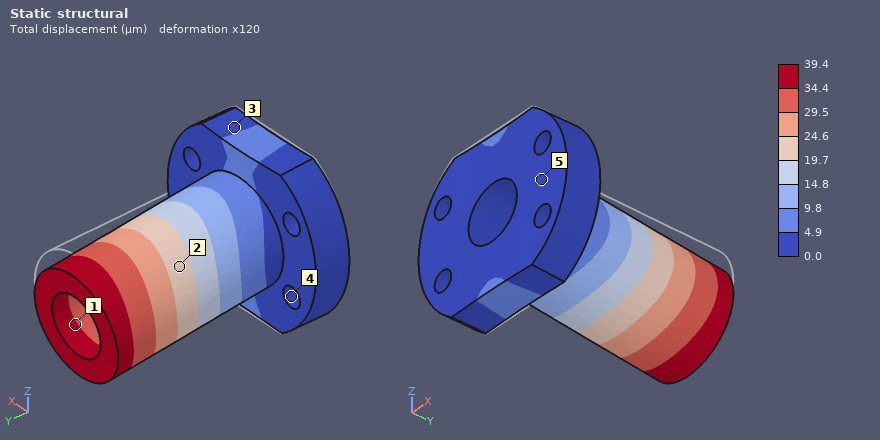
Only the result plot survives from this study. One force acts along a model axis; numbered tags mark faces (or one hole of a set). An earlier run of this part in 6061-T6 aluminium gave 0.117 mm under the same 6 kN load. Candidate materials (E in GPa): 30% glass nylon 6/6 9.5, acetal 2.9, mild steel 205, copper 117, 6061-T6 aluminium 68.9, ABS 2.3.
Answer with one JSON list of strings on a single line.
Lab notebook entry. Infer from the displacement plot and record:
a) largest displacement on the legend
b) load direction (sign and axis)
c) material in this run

["39.4 µm", "-Z", "mild steel"]
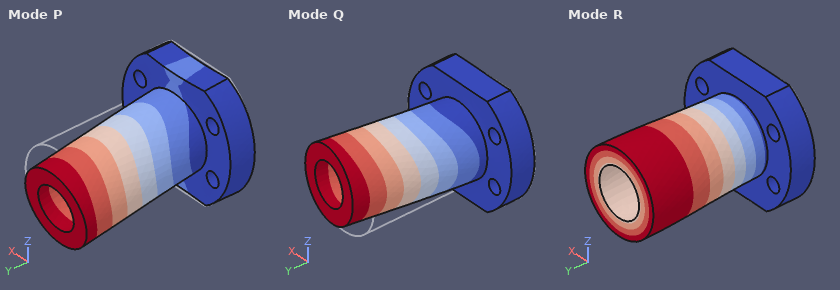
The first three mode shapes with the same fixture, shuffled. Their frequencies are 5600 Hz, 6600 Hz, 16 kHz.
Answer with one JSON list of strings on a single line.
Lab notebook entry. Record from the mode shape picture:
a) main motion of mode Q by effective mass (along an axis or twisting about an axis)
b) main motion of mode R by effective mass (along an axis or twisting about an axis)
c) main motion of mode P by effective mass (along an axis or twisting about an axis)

["along X", "twisting about Y", "along Z"]
